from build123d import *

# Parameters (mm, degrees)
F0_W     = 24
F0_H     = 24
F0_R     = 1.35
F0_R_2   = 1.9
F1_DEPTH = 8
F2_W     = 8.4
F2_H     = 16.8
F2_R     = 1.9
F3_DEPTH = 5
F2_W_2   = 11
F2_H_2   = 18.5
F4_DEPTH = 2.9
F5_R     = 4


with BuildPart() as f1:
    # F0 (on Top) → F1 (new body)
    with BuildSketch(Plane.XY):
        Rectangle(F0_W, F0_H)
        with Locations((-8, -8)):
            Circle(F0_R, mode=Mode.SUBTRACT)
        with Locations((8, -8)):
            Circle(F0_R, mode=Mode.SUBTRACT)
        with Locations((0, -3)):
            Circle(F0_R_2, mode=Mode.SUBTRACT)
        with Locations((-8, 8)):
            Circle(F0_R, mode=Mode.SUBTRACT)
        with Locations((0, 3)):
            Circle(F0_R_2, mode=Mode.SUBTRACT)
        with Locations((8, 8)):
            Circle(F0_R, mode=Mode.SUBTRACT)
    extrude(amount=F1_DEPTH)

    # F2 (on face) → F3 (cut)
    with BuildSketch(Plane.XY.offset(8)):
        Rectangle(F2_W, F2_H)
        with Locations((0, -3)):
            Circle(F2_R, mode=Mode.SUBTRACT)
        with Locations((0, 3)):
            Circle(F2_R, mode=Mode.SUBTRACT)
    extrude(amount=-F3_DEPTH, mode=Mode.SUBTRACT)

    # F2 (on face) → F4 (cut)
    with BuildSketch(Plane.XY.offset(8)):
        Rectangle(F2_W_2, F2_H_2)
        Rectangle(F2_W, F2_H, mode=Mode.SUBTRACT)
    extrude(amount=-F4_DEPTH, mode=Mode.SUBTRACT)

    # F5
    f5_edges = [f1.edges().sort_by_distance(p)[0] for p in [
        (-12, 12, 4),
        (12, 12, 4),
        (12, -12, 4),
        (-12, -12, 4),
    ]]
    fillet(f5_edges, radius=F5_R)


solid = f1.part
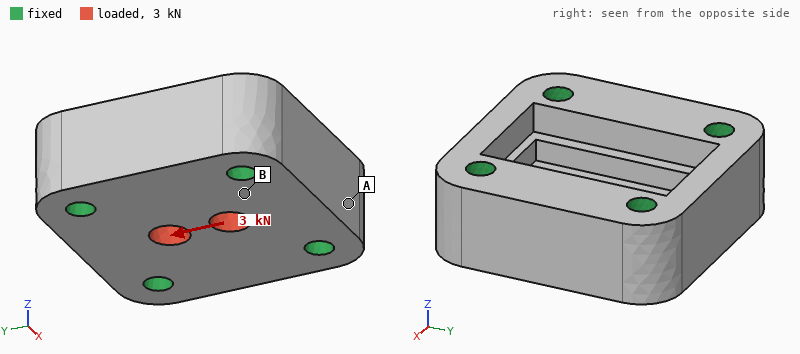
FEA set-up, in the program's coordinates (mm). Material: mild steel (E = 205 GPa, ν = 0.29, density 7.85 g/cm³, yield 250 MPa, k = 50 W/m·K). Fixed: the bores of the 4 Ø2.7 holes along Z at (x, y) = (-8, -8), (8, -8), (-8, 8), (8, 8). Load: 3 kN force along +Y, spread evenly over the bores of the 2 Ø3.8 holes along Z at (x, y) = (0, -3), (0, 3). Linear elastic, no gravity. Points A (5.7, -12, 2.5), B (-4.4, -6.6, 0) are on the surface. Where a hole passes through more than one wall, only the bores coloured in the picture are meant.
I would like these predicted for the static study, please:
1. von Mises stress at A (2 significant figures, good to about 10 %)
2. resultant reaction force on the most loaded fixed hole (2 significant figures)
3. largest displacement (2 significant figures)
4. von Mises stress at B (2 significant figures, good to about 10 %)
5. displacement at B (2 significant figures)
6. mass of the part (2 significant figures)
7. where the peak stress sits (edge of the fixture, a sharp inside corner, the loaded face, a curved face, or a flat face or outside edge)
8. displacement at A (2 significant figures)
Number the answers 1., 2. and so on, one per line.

1. 10 MPa
2. 820 N
3. 3.0 µm
4. 36 MPa
5. 0.72 µm
6. 26 g
7. the loaded face
8. 0.46 µm
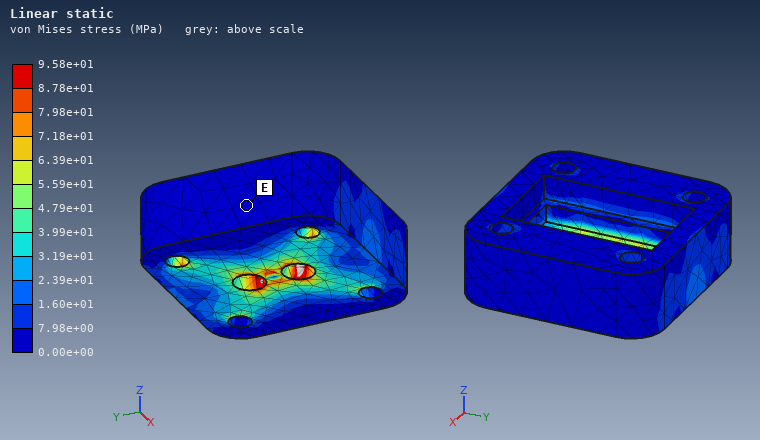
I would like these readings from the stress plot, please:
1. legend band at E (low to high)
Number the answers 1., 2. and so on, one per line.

1. 0.00e+00 to 7.98e+00 MPa
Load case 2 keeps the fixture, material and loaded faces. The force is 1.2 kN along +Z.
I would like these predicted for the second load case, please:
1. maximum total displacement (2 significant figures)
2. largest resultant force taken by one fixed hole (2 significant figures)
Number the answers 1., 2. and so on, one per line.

1. 3.8 µm
2. 330 N
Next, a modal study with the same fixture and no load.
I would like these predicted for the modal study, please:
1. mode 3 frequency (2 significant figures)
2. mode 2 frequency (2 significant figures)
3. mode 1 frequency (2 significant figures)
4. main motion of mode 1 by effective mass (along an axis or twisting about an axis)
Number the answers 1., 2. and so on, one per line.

1. 83 kHz
2. 80 kHz
3. 72 kHz
4. along Z
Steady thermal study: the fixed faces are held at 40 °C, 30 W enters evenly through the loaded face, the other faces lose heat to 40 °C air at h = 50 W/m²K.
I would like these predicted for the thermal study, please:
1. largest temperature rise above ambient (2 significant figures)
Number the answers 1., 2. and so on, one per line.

1. 49 K
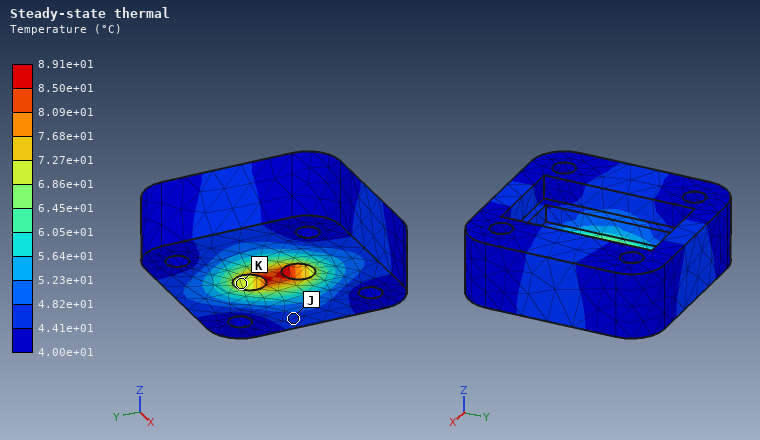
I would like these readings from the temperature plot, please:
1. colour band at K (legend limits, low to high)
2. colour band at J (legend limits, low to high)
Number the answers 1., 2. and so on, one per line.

1. 6.86e+01 to 7.27e+01 °C
2. 4.41e+01 to 4.82e+01 °C
